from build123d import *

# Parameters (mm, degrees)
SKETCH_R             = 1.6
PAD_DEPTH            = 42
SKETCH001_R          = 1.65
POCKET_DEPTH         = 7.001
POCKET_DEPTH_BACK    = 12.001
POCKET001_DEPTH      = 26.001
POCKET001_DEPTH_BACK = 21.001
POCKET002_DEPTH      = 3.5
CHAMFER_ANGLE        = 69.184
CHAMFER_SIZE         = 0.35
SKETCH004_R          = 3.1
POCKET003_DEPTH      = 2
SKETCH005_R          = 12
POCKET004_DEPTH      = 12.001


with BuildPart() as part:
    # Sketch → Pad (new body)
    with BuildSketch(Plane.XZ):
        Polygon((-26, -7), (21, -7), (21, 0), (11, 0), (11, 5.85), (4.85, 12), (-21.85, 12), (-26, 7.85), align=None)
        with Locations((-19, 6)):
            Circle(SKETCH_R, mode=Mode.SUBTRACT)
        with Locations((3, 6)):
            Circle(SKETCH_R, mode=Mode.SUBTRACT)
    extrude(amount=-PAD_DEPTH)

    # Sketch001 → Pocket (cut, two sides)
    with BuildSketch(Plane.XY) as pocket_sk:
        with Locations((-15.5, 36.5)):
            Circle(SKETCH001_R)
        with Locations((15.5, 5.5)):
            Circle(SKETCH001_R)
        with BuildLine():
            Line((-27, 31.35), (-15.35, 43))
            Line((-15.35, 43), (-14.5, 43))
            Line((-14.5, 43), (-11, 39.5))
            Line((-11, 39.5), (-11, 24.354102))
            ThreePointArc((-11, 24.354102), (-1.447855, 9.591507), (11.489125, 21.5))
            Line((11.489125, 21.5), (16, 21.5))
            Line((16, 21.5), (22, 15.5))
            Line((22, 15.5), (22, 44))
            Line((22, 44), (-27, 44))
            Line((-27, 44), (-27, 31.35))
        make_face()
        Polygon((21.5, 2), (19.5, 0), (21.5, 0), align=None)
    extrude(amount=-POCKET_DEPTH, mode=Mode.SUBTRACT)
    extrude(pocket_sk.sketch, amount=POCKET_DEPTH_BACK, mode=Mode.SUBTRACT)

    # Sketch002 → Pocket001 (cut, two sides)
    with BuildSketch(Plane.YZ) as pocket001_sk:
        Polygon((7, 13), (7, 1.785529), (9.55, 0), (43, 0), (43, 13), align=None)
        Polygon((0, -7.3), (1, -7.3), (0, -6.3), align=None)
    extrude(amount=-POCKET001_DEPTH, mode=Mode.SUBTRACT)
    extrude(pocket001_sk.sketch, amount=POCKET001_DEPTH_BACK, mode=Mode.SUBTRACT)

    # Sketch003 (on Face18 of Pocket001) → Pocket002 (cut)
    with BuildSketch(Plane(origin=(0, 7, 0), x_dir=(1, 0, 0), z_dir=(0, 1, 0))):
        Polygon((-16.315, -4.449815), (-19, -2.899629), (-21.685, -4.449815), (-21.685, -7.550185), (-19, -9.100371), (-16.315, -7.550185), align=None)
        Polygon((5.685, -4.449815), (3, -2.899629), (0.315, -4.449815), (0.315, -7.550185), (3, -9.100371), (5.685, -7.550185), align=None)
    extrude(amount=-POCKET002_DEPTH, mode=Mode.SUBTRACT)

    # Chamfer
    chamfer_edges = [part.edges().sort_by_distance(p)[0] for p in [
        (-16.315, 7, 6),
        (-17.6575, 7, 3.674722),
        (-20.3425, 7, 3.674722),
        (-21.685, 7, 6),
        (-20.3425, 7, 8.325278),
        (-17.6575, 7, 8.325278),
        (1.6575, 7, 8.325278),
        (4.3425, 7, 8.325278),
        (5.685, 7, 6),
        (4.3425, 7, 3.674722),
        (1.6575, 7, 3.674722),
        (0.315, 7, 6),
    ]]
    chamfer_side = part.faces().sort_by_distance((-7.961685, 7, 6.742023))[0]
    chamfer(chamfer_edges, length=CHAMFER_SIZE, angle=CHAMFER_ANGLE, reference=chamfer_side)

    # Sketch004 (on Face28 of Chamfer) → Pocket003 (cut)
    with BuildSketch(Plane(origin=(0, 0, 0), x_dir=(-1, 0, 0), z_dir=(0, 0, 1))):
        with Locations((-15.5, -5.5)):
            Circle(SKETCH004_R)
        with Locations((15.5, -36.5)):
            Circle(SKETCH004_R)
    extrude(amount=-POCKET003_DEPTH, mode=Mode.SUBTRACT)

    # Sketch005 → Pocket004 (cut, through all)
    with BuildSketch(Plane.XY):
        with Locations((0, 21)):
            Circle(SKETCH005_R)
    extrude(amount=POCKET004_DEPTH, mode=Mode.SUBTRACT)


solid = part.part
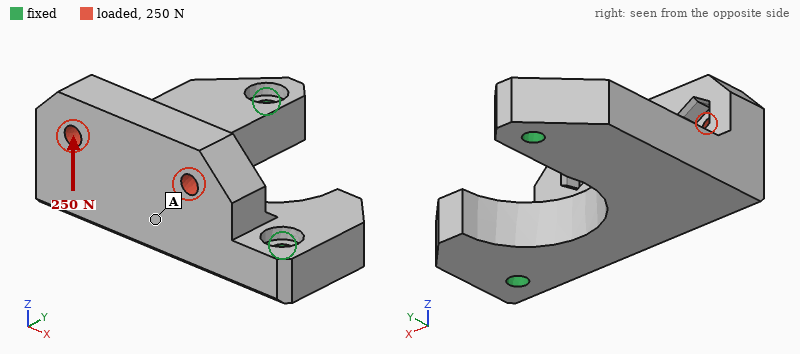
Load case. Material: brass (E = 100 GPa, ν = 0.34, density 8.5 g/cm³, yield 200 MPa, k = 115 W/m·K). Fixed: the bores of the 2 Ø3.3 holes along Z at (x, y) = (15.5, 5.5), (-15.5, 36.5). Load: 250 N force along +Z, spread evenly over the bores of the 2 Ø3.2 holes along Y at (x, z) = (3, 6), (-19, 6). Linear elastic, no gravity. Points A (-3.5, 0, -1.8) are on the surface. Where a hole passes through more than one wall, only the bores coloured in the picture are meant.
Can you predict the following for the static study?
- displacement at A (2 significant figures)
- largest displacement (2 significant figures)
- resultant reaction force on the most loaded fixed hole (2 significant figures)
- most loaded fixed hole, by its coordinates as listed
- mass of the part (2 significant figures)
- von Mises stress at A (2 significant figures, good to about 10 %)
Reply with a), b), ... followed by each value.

a) 15 µm
b) 34 µm
c) 170 N
d) (15.5, 5.5)
e) 83 g
f) 7.6 MPa
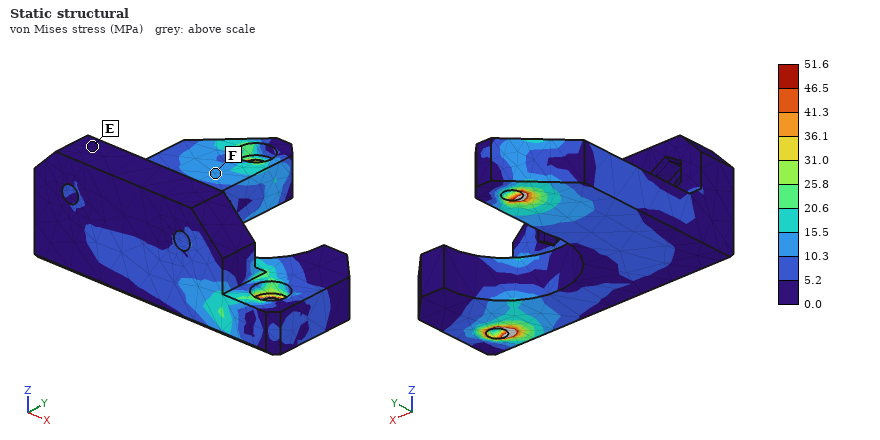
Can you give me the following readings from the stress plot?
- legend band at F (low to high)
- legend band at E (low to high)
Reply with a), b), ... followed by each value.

a) 10.3 to 15.5 MPa
b) 0.0 to 5.2 MPa
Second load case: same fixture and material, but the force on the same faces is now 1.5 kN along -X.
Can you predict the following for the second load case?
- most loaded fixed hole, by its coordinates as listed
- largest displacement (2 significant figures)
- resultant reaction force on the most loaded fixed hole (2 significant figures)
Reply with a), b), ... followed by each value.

a) (15.5, 5.5)
b) 84 µm
c) 1.5 kN
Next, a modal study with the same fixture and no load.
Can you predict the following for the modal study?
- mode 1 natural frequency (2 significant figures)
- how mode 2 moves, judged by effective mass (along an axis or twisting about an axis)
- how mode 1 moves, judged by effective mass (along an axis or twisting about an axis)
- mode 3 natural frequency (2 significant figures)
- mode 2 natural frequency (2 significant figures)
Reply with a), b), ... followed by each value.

a) 2400 Hz
b) along Y
c) along Z
d) 12 kHz
e) 7400 Hz
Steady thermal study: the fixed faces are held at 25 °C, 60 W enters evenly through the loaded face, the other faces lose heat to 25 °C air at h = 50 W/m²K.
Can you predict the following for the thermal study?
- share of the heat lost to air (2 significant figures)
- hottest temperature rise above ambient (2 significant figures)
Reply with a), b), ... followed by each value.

a) 13 %
b) 81 K
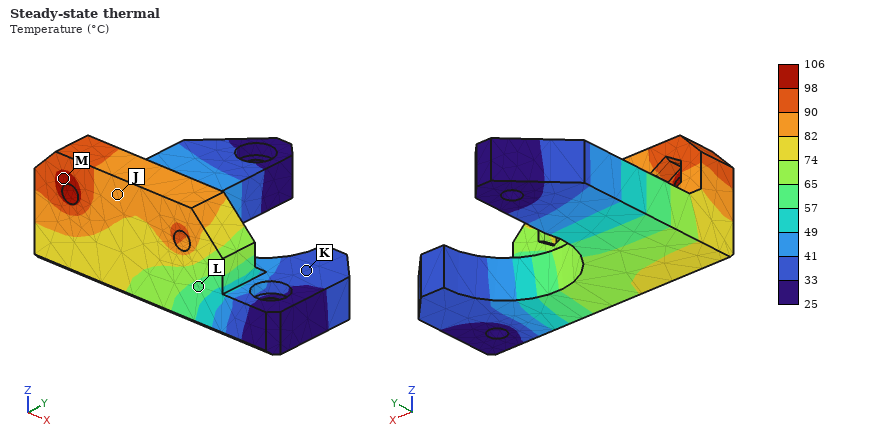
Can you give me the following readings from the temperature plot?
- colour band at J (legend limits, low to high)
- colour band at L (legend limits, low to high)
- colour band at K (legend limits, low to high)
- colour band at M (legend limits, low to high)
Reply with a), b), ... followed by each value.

a) 82 to 90 °C
b) 57 to 65 °C
c) 33 to 41 °C
d) 98 to 106 °C
